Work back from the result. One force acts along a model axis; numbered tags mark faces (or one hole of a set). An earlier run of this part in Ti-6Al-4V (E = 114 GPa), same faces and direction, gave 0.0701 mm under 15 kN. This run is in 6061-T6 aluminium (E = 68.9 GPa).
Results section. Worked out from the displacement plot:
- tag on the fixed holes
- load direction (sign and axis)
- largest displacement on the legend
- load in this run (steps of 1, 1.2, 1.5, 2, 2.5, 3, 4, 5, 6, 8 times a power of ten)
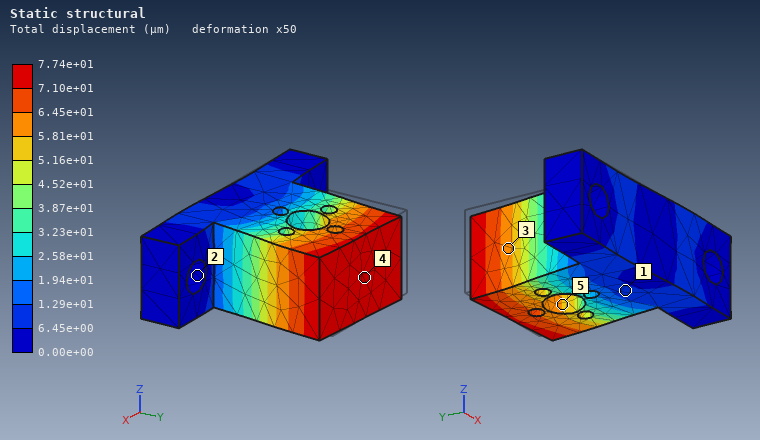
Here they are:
2
+X
7.74e+01 µm
10 kN
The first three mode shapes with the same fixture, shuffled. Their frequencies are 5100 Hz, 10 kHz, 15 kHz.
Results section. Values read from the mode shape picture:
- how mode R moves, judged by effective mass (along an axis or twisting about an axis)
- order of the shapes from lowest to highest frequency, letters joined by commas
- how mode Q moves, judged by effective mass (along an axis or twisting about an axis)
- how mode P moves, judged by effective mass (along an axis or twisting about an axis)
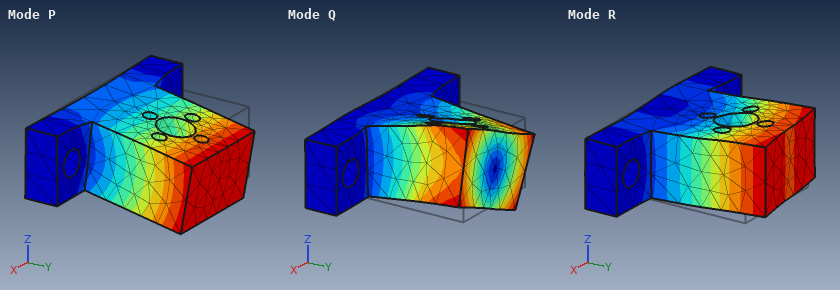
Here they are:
along X
P, R, Q
twisting about Y
along Z
